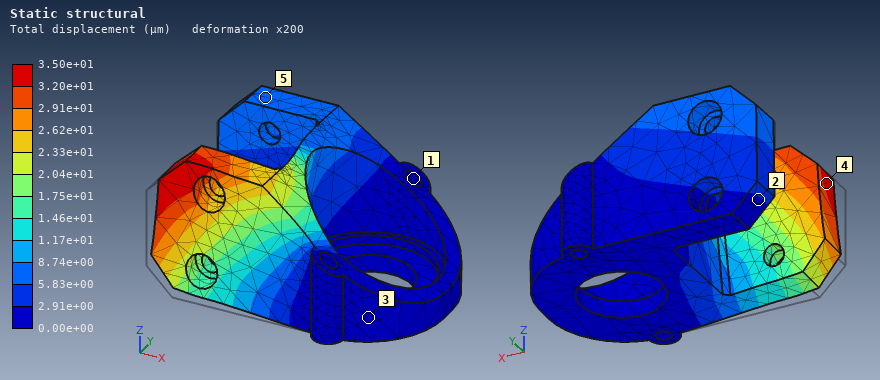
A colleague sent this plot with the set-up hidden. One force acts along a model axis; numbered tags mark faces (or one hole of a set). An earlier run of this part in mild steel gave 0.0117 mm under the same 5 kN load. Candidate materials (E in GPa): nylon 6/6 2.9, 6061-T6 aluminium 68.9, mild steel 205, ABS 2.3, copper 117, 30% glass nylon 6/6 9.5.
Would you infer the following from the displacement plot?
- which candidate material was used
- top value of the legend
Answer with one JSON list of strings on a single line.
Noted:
["6061-T6 aluminium", "3.50e+01 µm"]
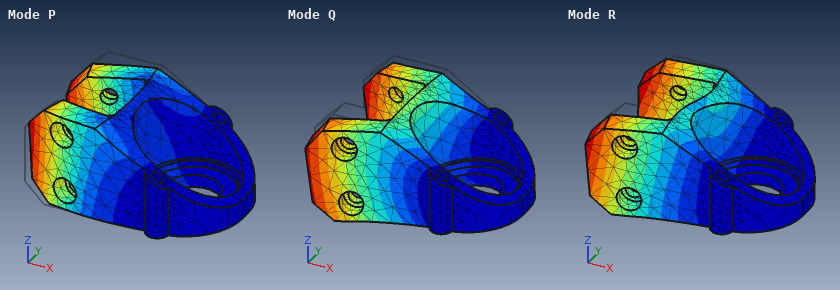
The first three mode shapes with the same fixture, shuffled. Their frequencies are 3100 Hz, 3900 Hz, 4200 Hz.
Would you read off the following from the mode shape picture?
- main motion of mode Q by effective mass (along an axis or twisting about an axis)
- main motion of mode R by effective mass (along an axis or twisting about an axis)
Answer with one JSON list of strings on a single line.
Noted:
["along Z", "along Y"]
